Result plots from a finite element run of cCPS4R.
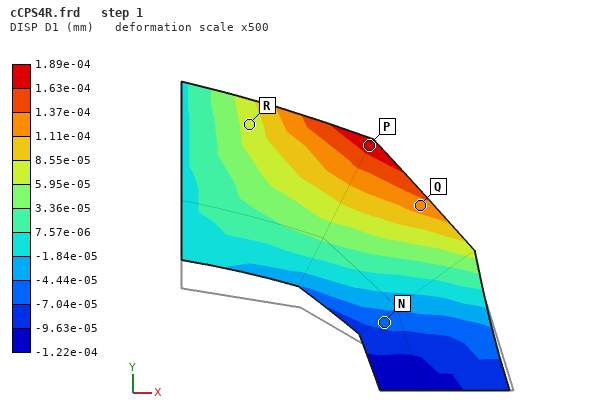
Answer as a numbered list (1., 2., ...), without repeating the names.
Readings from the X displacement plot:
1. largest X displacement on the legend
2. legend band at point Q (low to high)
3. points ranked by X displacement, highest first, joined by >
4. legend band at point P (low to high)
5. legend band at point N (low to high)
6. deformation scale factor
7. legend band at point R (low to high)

1. 1.89e-04 mm
2. 1.11e-04 to 1.37e-04 mm
3. P > Q > R > N
4. 1.63e-04 to 1.89e-04 mm
5. -7.04e-05 to -4.44e-05 mm
6. 500
7. 5.95e-05 to 8.55e-05 mm
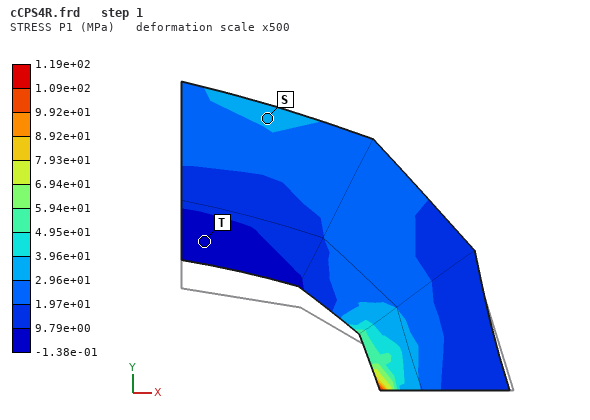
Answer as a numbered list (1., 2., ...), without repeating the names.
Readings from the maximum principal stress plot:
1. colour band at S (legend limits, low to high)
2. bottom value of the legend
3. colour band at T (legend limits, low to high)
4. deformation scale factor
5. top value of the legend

1. 2.96e+01 to 3.96e+01 MPa
2. -1.38e-01 MPa
3. -1.38e-01 to 9.79e+00 MPa
4. 500
5. 1.19e+02 MPa
